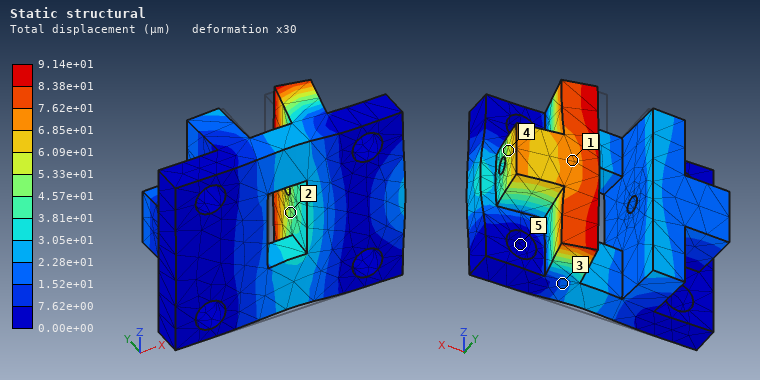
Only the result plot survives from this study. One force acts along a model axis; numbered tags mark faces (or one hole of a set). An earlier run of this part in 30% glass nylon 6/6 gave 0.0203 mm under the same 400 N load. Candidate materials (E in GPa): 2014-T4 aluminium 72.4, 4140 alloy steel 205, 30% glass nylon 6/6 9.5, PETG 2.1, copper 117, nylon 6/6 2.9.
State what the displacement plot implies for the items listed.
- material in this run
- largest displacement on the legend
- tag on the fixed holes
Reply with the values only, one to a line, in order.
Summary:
PETG
9.14e+01 µm
5
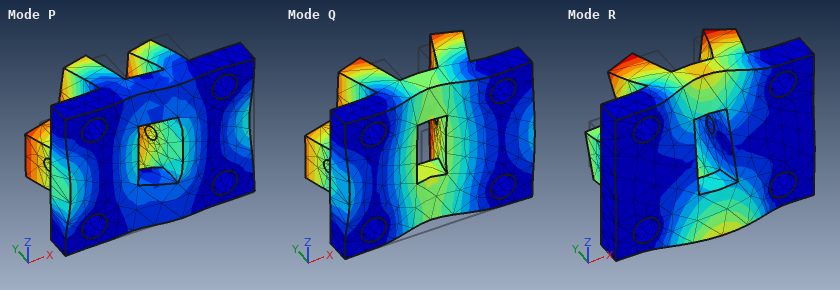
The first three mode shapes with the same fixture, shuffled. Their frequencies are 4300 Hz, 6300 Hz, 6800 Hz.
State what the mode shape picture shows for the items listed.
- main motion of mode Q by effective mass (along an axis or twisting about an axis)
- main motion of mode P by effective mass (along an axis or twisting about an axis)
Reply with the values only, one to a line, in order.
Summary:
along Y
along X
